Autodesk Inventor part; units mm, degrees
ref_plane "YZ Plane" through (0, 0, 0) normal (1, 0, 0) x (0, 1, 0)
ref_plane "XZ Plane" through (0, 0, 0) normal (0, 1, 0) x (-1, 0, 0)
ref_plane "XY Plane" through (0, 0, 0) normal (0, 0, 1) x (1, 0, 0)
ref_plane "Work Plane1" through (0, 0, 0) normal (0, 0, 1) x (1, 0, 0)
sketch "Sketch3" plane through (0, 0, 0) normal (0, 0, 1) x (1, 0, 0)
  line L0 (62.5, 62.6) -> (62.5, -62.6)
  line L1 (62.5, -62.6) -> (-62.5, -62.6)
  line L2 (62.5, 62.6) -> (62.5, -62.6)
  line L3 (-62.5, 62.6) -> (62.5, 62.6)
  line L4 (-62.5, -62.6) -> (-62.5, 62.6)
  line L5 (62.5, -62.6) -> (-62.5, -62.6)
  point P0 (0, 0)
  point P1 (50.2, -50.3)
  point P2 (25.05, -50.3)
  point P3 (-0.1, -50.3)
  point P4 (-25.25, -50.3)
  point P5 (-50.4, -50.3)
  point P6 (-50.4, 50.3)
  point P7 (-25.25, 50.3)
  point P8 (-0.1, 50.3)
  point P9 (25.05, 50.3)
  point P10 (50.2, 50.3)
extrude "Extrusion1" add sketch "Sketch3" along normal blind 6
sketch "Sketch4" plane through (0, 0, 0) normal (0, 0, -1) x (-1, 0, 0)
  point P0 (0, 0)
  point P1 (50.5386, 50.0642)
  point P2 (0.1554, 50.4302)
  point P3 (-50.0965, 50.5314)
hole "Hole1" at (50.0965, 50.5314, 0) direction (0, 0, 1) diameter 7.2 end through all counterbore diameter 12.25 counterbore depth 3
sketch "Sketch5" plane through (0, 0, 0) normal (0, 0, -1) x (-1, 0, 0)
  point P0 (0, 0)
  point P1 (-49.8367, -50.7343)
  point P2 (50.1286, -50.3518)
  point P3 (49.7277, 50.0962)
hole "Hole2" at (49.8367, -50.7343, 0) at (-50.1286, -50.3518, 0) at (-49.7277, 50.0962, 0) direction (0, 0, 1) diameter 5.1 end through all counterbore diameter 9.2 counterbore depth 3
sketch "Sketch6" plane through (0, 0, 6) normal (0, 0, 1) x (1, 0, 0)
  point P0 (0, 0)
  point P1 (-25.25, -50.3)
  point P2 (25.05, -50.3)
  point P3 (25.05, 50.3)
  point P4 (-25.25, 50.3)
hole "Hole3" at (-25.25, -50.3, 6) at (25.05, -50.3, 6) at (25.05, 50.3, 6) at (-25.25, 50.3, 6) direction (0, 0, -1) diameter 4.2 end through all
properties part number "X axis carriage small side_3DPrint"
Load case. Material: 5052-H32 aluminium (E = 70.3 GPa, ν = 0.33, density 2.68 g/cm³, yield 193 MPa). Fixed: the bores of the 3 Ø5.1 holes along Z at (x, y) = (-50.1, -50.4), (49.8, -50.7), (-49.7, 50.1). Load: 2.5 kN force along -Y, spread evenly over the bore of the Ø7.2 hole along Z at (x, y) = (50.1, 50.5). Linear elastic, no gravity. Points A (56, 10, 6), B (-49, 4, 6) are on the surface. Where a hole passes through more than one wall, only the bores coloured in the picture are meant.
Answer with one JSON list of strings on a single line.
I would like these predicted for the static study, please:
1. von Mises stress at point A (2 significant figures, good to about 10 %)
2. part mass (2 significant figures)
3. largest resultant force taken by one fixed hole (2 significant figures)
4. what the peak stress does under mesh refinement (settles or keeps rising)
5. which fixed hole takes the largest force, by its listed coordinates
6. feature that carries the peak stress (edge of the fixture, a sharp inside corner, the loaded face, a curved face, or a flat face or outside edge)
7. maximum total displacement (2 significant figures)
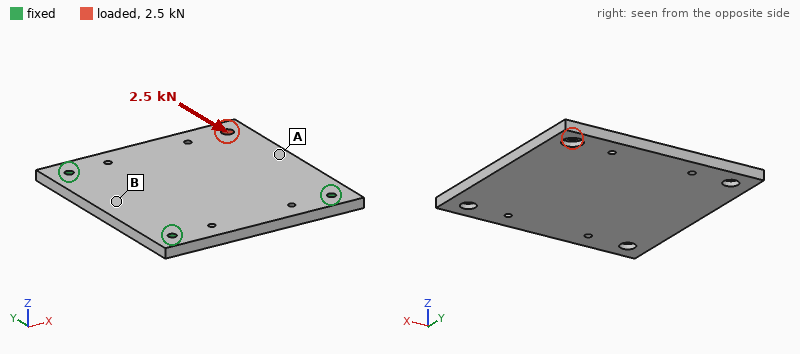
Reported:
["19 MPa", "250 g", "1.8 kN", "keeps rising", "(49.8, -50.7)", "edge of the fixture", "0.12 mm"]
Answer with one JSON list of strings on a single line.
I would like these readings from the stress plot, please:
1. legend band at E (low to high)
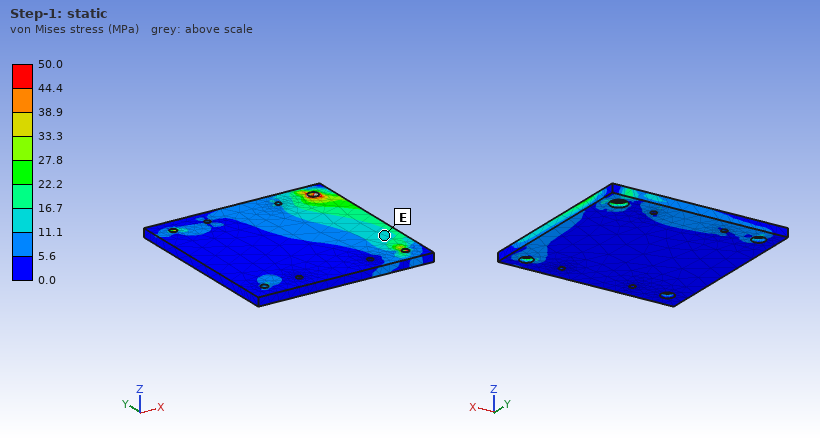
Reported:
["11.1 to 16.7 MPa"]
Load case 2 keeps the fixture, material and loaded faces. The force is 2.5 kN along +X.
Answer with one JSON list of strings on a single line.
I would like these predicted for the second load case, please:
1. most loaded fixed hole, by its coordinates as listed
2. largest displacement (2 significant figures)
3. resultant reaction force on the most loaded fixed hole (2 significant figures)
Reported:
["(-49.7, 50.1)", "0.12 mm", "1.8 kN"]
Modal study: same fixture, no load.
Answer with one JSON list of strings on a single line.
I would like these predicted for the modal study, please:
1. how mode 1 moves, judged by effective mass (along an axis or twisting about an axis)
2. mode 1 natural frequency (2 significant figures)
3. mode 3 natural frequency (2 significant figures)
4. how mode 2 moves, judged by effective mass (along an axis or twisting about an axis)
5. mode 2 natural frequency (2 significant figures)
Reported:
["along Z", "640 Hz", "2300 Hz", "along Z", "1900 Hz"]
